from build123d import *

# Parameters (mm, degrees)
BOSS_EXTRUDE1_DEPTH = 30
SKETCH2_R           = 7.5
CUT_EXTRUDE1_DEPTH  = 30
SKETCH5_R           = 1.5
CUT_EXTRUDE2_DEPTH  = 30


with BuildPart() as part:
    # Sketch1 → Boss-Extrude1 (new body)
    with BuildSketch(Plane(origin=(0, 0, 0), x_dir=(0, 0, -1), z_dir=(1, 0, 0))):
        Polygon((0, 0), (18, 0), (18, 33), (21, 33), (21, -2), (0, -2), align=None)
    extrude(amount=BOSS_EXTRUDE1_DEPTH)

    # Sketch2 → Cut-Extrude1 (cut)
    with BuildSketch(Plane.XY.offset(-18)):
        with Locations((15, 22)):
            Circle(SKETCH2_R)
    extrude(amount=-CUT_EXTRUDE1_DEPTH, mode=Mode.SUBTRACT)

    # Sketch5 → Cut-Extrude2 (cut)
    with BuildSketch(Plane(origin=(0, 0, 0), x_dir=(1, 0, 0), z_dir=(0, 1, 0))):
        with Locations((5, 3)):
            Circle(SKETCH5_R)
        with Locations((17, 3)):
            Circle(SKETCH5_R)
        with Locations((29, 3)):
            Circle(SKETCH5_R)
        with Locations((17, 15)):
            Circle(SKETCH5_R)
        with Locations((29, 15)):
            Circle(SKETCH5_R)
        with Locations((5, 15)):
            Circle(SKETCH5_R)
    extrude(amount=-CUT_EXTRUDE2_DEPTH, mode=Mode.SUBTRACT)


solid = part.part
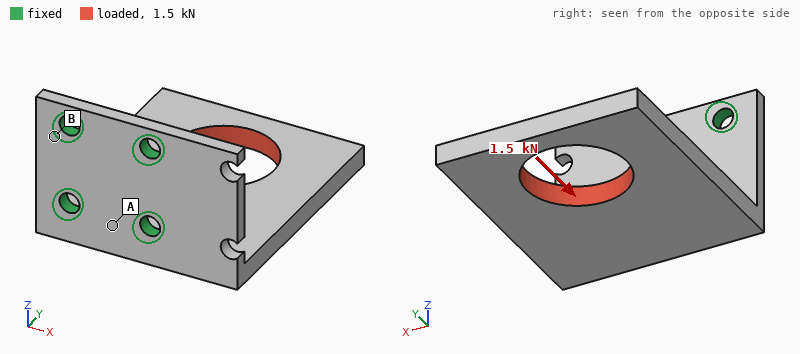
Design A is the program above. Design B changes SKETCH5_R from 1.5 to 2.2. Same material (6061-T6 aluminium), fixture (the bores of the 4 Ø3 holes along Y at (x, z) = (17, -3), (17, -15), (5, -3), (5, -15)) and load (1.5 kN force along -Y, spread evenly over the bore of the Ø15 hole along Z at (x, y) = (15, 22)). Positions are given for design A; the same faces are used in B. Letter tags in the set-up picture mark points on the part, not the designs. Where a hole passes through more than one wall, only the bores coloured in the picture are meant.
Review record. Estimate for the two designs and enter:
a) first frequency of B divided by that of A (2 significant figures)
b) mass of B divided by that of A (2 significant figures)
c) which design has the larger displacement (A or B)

1.1
0.98
A
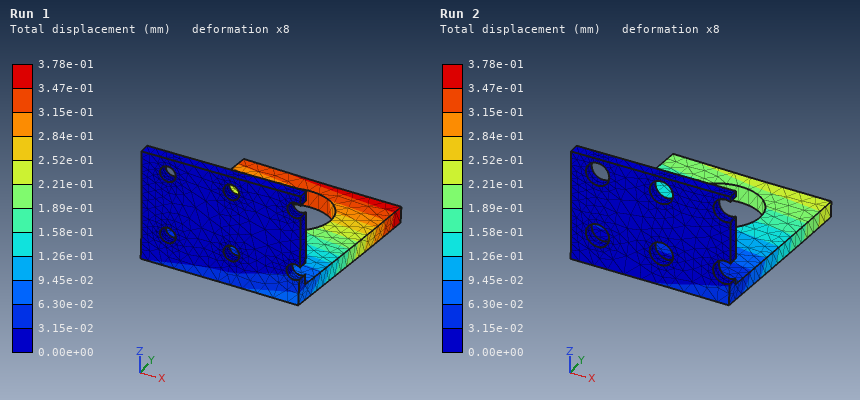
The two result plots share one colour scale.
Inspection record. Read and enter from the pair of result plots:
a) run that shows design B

Run 2
